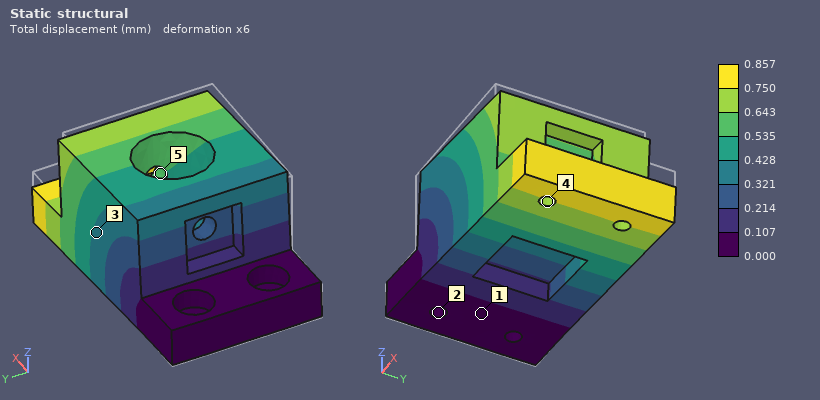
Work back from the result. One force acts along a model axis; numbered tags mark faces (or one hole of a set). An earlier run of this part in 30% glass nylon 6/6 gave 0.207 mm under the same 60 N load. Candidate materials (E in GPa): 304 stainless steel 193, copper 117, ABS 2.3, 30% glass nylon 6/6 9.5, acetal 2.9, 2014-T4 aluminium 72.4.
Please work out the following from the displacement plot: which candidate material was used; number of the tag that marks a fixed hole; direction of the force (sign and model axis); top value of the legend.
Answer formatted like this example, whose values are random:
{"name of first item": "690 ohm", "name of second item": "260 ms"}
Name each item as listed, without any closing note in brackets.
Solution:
{"which candidate material was used": "ABS", "number of the tag that marks a fixed hole": "2", "direction of the force": "-Z", "top value of the legend": "0.857 mm"}
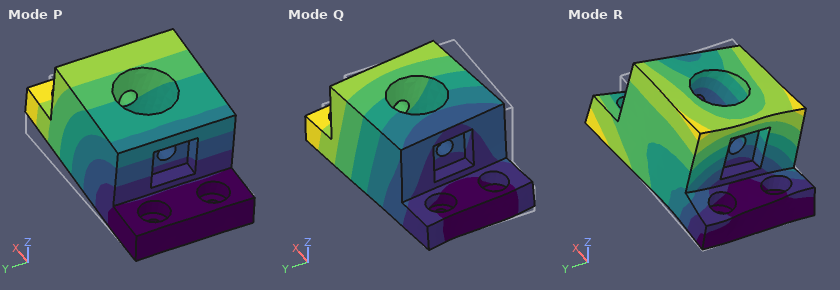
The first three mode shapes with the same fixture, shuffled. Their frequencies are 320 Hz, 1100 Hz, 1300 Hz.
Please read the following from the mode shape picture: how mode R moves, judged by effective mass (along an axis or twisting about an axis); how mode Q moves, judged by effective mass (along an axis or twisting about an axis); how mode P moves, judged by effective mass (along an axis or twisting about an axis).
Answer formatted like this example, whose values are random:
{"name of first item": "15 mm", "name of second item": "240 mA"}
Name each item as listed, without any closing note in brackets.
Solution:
{"how mode R moves, judged by effective mass": "twisting about X", "how mode Q moves, judged by effective mass": "along Y", "how mode P moves, judged by effective mass": "along Z"}
